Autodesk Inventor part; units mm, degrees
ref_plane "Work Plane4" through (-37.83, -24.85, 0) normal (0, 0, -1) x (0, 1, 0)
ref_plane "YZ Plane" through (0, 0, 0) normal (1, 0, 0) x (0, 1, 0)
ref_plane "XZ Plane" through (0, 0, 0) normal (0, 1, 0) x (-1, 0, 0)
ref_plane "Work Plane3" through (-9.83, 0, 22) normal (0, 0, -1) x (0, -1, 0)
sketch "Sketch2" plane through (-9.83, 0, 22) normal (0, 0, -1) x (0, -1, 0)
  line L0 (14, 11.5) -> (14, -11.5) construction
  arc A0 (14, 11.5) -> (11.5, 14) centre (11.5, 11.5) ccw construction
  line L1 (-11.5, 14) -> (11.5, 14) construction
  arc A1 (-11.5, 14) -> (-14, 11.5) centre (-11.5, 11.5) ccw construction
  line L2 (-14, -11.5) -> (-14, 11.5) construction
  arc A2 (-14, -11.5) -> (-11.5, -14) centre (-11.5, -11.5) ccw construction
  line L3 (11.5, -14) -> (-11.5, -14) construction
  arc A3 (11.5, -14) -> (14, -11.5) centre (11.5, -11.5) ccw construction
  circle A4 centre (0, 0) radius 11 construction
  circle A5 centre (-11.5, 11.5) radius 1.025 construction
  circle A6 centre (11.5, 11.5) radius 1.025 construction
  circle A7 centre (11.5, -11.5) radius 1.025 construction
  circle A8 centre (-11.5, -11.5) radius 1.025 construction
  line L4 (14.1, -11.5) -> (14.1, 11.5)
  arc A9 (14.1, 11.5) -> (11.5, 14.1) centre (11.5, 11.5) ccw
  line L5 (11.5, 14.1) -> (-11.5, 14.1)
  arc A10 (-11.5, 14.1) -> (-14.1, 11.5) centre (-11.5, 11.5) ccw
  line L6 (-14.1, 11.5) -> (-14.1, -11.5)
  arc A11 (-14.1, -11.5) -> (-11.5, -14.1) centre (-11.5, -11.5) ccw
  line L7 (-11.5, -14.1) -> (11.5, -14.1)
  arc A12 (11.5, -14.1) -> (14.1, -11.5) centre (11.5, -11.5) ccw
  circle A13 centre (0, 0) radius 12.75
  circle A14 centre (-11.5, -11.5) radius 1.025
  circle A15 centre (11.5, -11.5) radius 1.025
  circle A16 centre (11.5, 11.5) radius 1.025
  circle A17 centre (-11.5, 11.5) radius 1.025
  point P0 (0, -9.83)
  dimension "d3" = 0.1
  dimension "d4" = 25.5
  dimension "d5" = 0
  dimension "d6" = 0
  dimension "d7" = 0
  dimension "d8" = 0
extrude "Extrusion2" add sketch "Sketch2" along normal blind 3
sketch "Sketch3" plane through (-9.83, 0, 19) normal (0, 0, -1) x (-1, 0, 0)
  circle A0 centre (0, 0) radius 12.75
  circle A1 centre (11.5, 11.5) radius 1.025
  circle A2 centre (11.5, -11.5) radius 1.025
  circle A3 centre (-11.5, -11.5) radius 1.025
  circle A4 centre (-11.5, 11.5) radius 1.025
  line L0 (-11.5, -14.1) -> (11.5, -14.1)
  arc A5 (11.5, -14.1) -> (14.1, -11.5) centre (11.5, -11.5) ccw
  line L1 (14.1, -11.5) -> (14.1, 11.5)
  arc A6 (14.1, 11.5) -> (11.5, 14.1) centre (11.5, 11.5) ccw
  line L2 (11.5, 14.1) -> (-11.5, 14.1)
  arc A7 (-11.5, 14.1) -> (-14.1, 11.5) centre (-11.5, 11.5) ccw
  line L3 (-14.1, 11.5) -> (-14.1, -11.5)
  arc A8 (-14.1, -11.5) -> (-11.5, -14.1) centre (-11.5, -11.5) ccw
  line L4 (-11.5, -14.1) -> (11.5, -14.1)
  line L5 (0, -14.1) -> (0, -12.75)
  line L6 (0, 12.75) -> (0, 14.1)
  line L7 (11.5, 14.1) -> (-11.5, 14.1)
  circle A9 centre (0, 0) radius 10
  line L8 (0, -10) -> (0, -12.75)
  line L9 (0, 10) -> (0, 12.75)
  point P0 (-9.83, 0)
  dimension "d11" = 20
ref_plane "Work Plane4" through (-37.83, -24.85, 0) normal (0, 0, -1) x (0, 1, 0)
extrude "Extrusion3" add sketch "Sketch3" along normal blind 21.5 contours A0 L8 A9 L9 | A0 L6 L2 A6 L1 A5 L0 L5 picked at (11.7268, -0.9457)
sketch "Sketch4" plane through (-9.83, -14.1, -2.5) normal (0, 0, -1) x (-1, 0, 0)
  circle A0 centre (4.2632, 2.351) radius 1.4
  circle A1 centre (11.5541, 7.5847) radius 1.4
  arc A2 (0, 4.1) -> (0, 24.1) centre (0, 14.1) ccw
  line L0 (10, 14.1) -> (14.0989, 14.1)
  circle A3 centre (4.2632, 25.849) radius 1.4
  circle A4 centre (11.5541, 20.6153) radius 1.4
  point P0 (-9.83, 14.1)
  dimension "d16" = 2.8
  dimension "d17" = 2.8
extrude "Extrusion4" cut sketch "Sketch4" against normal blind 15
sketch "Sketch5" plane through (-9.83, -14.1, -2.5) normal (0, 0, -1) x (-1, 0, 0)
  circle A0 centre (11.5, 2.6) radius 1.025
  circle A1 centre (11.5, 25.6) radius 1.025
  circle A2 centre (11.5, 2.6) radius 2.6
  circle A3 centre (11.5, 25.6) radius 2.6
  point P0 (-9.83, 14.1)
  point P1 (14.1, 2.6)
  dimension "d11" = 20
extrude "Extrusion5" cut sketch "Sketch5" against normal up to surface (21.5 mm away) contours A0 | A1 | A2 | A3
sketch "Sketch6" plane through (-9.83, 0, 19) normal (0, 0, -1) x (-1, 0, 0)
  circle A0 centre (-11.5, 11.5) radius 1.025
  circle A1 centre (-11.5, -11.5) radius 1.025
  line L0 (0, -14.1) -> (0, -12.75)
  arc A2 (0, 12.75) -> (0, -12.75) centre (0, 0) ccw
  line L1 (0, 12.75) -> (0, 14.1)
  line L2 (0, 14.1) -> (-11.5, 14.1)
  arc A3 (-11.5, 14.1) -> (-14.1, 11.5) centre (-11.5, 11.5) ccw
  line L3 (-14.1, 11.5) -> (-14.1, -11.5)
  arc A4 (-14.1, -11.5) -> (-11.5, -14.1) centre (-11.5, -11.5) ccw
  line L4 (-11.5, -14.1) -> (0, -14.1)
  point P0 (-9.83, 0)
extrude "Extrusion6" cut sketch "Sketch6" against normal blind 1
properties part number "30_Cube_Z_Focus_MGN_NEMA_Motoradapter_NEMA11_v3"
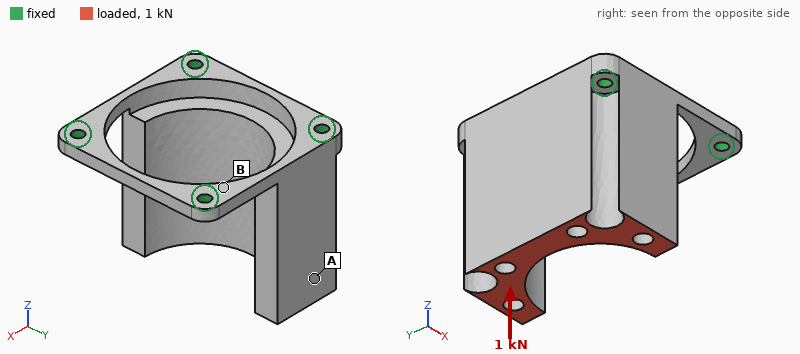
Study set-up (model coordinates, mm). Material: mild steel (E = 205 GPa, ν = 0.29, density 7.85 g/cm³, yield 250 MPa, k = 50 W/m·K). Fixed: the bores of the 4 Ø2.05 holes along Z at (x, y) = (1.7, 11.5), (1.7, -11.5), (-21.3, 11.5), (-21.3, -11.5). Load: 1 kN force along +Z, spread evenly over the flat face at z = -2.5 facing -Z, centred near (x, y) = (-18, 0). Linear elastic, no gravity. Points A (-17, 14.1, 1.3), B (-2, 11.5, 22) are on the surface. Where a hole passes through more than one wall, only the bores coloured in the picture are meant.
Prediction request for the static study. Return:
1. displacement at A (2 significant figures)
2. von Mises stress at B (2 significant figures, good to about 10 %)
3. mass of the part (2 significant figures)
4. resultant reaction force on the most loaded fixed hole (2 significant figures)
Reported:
12 µm
31 MPa
35 g
490 N
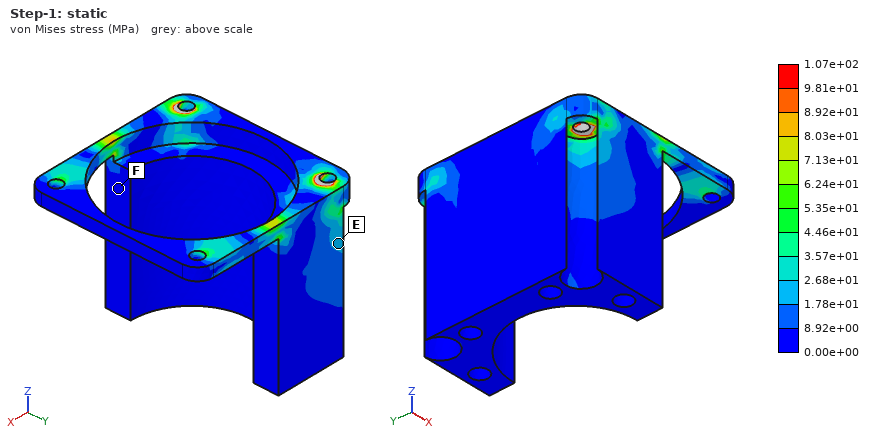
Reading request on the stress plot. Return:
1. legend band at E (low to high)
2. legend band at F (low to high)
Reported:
1.78e+01 to 2.68e+01 MPa
0.00e+00 to 8.92e+00 MPa
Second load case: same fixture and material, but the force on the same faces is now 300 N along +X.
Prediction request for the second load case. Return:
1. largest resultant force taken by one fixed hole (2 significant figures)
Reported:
210 N
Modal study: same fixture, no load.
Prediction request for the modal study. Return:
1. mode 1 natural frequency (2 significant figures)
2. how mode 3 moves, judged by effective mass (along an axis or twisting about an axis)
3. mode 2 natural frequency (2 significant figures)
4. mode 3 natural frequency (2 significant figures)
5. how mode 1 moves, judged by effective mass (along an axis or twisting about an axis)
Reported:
4100 Hz
along Y
8800 Hz
14 kHz
along X
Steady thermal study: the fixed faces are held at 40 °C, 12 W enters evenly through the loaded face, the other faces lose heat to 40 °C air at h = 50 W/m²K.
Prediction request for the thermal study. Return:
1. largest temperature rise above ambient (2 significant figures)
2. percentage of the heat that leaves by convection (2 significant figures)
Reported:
37 K
32 %
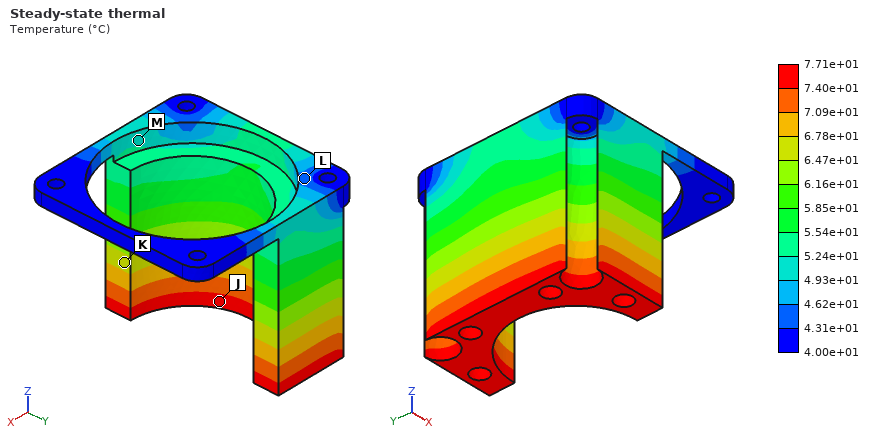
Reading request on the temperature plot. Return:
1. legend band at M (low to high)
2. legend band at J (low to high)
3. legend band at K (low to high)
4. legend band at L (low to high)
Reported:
4.93e+01 to 5.24e+01 °C
7.40e+01 to 7.71e+01 °C
6.47e+01 to 6.78e+01 °C
4.31e+01 to 4.62e+01 °C
